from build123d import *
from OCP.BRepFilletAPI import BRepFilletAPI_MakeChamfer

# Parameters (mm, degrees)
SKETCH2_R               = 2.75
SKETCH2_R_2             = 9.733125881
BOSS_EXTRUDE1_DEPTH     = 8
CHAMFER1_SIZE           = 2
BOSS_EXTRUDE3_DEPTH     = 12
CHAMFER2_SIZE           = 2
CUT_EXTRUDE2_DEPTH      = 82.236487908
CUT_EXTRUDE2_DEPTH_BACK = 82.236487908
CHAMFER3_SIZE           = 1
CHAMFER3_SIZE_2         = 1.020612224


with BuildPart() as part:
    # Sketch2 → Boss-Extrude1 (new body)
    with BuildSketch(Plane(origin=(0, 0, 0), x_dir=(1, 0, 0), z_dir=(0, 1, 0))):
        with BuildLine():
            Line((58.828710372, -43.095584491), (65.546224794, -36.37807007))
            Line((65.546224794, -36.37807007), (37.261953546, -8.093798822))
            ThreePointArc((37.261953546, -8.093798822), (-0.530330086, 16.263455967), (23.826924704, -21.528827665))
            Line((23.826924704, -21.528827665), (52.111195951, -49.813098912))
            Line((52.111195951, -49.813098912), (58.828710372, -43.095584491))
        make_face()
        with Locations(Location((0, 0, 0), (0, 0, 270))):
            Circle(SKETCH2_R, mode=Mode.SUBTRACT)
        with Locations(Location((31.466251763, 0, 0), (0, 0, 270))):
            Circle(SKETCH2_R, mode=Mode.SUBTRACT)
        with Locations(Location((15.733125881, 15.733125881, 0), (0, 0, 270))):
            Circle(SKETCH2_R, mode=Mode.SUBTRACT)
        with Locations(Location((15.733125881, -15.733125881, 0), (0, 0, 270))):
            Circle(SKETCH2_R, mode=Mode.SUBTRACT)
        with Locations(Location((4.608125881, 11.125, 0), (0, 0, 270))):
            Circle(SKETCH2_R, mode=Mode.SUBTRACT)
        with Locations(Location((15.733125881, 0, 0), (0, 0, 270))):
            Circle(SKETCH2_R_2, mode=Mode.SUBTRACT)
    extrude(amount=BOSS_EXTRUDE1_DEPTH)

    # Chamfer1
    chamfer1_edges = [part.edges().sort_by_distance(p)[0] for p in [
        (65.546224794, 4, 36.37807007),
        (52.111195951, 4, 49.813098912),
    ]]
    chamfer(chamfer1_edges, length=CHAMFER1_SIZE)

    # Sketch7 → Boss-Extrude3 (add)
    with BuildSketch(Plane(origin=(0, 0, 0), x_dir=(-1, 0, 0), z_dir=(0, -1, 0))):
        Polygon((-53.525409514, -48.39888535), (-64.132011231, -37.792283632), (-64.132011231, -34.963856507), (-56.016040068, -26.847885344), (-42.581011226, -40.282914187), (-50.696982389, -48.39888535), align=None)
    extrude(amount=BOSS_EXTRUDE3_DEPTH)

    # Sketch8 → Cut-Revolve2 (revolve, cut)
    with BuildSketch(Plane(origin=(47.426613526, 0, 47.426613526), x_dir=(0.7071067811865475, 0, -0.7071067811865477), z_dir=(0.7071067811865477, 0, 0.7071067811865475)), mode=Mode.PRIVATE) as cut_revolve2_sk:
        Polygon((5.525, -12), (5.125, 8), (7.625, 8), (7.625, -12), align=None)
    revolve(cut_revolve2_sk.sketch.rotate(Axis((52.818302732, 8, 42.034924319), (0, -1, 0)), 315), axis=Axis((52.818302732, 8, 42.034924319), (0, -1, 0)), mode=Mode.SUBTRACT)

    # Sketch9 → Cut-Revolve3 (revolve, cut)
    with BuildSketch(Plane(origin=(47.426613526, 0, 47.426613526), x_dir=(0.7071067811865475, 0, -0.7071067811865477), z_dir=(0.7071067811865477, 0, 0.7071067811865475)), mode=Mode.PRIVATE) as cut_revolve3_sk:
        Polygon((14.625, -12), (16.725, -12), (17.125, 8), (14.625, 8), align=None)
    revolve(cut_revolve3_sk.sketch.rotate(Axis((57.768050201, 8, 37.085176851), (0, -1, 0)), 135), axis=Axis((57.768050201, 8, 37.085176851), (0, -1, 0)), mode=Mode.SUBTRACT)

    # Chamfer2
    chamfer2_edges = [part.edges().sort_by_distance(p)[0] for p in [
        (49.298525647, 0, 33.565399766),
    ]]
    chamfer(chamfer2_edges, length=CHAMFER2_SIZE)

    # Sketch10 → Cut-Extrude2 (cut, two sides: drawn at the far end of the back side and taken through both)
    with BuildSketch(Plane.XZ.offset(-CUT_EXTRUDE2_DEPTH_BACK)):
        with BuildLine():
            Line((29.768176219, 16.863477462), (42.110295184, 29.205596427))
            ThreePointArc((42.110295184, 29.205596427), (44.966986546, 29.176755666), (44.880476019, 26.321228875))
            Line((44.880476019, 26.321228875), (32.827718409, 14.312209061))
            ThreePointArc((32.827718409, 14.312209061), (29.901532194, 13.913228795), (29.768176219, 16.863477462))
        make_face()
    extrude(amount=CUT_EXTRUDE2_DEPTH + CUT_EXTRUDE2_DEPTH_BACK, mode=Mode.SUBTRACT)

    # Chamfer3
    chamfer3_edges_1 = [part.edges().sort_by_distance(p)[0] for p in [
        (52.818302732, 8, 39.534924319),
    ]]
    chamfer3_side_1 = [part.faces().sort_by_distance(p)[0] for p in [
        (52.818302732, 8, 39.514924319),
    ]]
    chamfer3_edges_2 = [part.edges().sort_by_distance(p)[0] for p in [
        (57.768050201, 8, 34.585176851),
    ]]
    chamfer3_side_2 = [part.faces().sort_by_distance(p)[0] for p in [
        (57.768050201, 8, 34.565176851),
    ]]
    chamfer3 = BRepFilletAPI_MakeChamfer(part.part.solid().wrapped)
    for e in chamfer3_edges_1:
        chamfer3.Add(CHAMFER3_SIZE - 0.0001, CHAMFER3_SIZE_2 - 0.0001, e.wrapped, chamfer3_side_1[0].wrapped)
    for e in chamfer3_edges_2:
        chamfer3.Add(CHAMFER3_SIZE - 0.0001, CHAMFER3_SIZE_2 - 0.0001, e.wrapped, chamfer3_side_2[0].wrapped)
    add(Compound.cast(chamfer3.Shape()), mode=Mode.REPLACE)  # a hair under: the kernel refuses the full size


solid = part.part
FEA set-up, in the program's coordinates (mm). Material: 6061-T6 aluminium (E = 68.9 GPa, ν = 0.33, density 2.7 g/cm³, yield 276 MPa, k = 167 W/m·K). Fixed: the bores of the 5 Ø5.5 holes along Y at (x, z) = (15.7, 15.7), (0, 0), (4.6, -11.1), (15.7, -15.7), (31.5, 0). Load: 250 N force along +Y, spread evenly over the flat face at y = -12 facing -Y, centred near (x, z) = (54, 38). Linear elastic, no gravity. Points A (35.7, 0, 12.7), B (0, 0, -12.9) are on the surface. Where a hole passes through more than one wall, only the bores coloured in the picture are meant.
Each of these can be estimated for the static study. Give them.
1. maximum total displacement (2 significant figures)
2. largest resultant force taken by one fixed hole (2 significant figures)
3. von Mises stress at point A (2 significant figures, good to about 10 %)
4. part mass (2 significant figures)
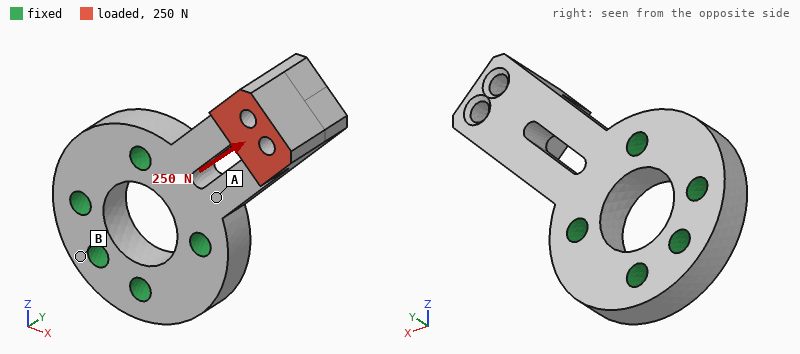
0.17 mm
140 N
44 MPa
47 g
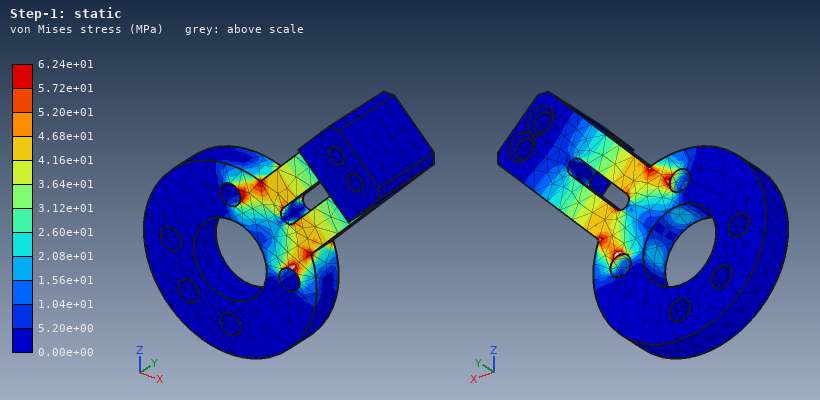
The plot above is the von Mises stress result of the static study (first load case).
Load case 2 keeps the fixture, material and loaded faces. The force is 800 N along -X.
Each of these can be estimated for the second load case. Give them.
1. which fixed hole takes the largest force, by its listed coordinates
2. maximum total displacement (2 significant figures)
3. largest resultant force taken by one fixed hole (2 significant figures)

(15.7, 15.7)
0.32 mm
1.4 kN
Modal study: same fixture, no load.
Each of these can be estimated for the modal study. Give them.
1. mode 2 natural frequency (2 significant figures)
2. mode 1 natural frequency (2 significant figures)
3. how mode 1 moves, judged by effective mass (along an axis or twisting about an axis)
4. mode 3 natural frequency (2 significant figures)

3800 Hz
1900 Hz
along Y
6700 Hz
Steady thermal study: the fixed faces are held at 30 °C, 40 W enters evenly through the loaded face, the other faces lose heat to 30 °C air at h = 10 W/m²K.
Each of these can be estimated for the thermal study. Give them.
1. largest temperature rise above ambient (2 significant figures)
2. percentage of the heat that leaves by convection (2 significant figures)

81 K
4.9 %
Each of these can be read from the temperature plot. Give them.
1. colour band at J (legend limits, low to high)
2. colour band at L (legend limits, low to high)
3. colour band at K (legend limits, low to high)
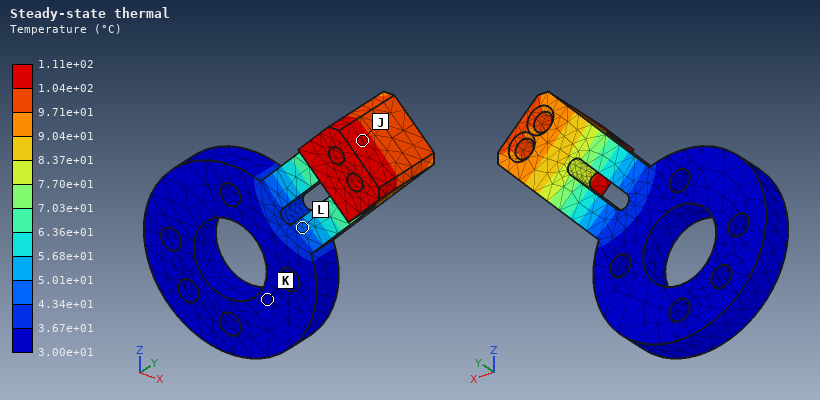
1.04e+02 to 1.11e+02 °C
4.34e+01 to 5.01e+01 °C
3.00e+01 to 3.67e+01 °C
